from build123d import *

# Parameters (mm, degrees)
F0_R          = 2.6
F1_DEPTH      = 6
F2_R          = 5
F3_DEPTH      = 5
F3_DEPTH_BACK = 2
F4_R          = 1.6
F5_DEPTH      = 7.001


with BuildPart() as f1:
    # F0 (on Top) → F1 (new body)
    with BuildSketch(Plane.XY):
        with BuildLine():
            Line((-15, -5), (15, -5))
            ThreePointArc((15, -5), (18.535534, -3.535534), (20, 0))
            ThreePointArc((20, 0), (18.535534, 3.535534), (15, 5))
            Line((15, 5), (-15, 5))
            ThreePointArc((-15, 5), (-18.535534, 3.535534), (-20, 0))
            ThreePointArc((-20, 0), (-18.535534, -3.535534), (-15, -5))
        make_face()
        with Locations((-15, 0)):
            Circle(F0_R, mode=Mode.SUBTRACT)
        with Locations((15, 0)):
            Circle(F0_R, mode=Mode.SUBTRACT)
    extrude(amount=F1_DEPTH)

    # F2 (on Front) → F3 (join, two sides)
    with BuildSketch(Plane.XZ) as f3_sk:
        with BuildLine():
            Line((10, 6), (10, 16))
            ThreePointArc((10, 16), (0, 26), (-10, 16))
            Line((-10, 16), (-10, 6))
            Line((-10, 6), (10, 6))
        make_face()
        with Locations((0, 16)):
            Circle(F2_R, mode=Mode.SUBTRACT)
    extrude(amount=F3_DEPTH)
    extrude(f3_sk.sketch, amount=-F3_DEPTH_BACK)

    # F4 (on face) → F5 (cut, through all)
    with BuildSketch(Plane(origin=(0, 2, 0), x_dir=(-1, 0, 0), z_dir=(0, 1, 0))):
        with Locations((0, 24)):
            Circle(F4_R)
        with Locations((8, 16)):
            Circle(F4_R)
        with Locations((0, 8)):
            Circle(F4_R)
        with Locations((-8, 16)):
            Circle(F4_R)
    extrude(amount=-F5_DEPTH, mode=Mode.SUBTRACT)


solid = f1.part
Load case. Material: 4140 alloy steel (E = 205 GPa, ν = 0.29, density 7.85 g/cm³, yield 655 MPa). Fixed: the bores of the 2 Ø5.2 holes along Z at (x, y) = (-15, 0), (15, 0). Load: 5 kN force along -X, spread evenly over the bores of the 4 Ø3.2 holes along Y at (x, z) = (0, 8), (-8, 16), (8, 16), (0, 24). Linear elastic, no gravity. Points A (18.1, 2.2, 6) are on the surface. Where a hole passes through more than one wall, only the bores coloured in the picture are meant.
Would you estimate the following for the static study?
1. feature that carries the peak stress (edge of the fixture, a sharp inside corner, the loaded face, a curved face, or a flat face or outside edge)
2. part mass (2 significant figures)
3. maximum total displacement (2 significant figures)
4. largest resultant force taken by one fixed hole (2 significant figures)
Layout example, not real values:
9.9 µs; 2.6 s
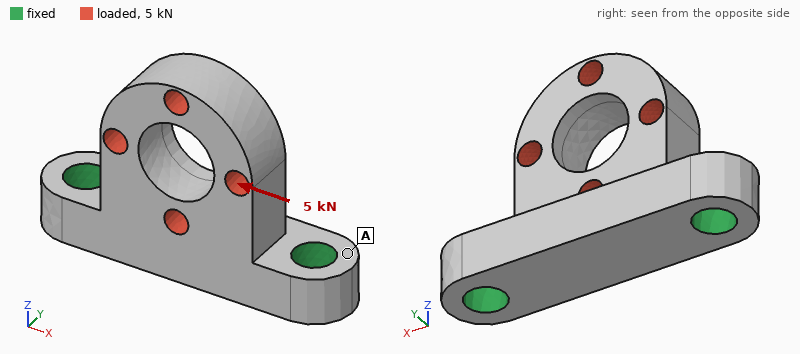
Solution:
the loaded face; 29 g; 48 µm; 3.7 kN
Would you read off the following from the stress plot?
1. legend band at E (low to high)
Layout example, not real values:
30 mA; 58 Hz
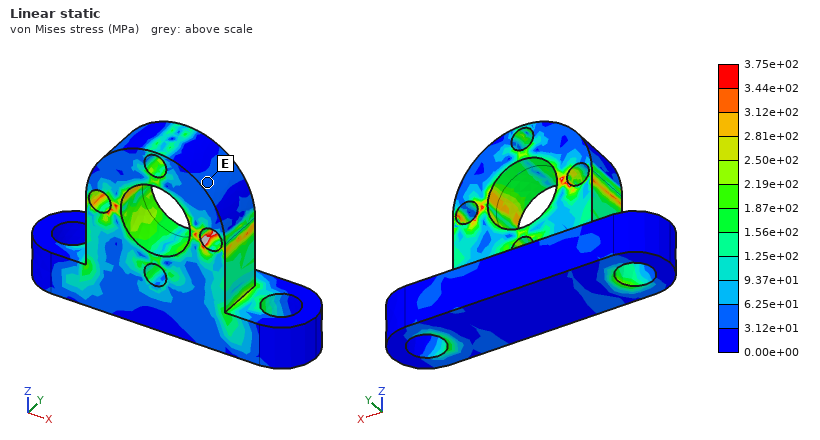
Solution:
3.12e+01 to 6.25e+01 MPa
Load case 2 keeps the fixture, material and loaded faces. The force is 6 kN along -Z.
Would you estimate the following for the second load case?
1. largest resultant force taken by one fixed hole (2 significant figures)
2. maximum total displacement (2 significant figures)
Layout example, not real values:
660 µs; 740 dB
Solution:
3.1 kN; 21 µm
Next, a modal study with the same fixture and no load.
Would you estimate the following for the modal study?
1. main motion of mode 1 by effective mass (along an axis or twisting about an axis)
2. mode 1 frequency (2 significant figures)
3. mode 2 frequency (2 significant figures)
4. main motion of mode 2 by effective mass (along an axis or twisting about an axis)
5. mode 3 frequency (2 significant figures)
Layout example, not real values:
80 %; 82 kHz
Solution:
along Y; 8900 Hz; 17 kHz; along X; 22 kHz
